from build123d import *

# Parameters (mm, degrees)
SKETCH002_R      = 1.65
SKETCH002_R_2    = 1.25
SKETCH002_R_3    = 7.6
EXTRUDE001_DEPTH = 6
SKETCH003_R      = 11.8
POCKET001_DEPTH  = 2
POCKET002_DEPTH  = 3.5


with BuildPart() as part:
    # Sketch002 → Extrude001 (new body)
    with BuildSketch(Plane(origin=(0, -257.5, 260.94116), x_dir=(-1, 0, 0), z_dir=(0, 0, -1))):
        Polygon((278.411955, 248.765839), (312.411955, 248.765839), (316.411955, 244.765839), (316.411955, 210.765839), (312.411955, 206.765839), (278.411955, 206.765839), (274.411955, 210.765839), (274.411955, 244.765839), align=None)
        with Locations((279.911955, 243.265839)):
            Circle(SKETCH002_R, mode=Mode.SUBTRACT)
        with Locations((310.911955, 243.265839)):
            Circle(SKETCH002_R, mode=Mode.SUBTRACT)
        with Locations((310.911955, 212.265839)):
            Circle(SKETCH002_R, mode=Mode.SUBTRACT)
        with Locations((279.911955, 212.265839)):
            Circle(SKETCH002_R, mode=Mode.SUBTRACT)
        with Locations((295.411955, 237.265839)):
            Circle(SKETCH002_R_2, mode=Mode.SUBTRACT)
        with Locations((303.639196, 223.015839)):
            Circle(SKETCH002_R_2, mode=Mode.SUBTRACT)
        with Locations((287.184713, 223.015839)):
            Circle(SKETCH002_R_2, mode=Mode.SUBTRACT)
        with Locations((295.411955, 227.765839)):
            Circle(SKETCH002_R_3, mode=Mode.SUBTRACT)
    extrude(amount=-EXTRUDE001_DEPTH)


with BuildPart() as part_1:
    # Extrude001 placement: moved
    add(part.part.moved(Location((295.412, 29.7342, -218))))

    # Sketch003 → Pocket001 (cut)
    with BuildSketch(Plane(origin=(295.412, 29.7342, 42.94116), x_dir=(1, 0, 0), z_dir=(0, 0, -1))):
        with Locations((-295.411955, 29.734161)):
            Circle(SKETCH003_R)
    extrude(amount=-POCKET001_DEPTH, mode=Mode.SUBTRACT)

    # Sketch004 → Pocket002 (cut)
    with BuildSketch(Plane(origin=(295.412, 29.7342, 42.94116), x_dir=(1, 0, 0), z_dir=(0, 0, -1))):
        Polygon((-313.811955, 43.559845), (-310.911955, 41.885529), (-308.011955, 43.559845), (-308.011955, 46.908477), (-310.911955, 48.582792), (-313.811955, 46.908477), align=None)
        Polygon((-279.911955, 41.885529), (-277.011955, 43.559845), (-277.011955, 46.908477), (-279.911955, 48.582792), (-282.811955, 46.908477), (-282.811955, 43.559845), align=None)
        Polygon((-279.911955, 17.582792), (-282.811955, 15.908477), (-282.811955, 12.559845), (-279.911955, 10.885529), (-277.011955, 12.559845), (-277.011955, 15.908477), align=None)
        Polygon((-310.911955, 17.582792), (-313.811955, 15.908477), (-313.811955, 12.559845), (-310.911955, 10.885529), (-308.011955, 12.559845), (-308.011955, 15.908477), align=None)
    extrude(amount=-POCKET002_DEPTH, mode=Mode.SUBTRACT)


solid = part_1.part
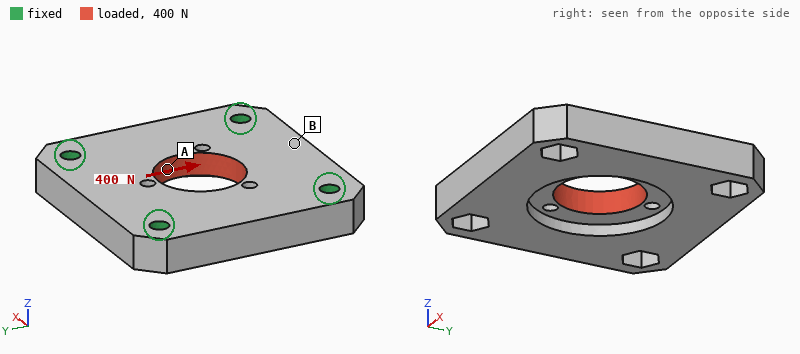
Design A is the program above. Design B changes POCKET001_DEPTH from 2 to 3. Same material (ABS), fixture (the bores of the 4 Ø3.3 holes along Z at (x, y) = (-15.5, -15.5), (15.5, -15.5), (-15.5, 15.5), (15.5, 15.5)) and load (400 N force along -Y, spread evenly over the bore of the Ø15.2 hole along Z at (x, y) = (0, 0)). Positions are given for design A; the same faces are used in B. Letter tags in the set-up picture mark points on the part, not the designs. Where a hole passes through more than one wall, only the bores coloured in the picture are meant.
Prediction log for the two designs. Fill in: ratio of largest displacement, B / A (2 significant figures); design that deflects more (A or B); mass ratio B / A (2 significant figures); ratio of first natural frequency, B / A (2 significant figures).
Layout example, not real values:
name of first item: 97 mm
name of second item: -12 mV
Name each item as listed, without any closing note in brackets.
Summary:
ratio of largest displacement, B / A: 1.2
design that deflects more: B
mass ratio B / A: 0.97
ratio of first natural frequency, B / A: 1.0
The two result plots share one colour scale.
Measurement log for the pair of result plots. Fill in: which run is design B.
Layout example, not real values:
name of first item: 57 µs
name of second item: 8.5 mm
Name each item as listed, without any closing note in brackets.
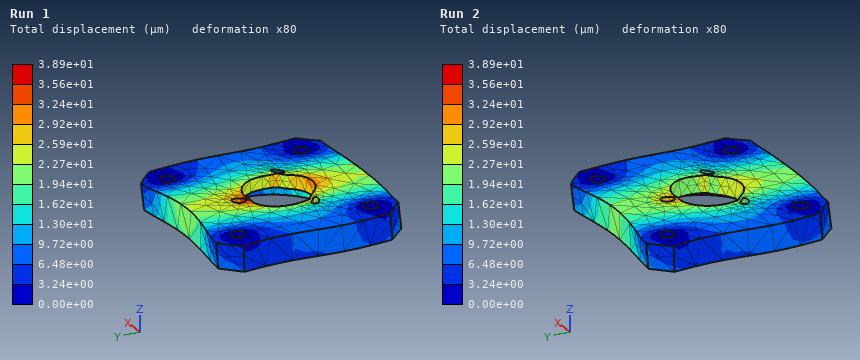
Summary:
which run is design B: Run 1
